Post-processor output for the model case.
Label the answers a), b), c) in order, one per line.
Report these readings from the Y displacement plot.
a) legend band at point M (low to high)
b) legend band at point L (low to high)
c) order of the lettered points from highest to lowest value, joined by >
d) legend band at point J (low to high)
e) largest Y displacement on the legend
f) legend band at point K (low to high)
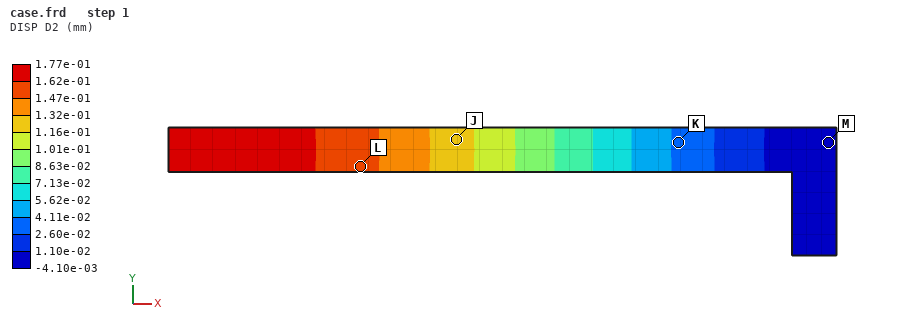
a) -4.10e-03 to 1.10e-02 mm
b) 1.47e-01 to 1.62e-01 mm
c) L > J > K > M
d) 1.16e-01 to 1.32e-01 mm
e) 1.77e-01 mm
f) 2.60e-02 to 4.11e-02 mm
